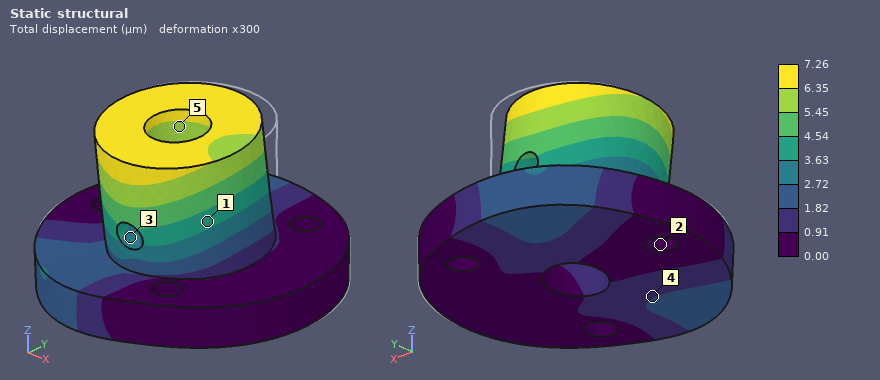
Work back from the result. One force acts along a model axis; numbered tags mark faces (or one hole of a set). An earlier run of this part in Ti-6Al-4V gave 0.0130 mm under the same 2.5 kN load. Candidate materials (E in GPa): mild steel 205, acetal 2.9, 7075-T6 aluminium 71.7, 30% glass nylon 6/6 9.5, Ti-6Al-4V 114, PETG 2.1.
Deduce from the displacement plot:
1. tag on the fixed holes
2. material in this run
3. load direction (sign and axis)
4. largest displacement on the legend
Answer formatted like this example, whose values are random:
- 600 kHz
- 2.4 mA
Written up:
- 2
- mild steel
- -Y
- 7.26 µm
